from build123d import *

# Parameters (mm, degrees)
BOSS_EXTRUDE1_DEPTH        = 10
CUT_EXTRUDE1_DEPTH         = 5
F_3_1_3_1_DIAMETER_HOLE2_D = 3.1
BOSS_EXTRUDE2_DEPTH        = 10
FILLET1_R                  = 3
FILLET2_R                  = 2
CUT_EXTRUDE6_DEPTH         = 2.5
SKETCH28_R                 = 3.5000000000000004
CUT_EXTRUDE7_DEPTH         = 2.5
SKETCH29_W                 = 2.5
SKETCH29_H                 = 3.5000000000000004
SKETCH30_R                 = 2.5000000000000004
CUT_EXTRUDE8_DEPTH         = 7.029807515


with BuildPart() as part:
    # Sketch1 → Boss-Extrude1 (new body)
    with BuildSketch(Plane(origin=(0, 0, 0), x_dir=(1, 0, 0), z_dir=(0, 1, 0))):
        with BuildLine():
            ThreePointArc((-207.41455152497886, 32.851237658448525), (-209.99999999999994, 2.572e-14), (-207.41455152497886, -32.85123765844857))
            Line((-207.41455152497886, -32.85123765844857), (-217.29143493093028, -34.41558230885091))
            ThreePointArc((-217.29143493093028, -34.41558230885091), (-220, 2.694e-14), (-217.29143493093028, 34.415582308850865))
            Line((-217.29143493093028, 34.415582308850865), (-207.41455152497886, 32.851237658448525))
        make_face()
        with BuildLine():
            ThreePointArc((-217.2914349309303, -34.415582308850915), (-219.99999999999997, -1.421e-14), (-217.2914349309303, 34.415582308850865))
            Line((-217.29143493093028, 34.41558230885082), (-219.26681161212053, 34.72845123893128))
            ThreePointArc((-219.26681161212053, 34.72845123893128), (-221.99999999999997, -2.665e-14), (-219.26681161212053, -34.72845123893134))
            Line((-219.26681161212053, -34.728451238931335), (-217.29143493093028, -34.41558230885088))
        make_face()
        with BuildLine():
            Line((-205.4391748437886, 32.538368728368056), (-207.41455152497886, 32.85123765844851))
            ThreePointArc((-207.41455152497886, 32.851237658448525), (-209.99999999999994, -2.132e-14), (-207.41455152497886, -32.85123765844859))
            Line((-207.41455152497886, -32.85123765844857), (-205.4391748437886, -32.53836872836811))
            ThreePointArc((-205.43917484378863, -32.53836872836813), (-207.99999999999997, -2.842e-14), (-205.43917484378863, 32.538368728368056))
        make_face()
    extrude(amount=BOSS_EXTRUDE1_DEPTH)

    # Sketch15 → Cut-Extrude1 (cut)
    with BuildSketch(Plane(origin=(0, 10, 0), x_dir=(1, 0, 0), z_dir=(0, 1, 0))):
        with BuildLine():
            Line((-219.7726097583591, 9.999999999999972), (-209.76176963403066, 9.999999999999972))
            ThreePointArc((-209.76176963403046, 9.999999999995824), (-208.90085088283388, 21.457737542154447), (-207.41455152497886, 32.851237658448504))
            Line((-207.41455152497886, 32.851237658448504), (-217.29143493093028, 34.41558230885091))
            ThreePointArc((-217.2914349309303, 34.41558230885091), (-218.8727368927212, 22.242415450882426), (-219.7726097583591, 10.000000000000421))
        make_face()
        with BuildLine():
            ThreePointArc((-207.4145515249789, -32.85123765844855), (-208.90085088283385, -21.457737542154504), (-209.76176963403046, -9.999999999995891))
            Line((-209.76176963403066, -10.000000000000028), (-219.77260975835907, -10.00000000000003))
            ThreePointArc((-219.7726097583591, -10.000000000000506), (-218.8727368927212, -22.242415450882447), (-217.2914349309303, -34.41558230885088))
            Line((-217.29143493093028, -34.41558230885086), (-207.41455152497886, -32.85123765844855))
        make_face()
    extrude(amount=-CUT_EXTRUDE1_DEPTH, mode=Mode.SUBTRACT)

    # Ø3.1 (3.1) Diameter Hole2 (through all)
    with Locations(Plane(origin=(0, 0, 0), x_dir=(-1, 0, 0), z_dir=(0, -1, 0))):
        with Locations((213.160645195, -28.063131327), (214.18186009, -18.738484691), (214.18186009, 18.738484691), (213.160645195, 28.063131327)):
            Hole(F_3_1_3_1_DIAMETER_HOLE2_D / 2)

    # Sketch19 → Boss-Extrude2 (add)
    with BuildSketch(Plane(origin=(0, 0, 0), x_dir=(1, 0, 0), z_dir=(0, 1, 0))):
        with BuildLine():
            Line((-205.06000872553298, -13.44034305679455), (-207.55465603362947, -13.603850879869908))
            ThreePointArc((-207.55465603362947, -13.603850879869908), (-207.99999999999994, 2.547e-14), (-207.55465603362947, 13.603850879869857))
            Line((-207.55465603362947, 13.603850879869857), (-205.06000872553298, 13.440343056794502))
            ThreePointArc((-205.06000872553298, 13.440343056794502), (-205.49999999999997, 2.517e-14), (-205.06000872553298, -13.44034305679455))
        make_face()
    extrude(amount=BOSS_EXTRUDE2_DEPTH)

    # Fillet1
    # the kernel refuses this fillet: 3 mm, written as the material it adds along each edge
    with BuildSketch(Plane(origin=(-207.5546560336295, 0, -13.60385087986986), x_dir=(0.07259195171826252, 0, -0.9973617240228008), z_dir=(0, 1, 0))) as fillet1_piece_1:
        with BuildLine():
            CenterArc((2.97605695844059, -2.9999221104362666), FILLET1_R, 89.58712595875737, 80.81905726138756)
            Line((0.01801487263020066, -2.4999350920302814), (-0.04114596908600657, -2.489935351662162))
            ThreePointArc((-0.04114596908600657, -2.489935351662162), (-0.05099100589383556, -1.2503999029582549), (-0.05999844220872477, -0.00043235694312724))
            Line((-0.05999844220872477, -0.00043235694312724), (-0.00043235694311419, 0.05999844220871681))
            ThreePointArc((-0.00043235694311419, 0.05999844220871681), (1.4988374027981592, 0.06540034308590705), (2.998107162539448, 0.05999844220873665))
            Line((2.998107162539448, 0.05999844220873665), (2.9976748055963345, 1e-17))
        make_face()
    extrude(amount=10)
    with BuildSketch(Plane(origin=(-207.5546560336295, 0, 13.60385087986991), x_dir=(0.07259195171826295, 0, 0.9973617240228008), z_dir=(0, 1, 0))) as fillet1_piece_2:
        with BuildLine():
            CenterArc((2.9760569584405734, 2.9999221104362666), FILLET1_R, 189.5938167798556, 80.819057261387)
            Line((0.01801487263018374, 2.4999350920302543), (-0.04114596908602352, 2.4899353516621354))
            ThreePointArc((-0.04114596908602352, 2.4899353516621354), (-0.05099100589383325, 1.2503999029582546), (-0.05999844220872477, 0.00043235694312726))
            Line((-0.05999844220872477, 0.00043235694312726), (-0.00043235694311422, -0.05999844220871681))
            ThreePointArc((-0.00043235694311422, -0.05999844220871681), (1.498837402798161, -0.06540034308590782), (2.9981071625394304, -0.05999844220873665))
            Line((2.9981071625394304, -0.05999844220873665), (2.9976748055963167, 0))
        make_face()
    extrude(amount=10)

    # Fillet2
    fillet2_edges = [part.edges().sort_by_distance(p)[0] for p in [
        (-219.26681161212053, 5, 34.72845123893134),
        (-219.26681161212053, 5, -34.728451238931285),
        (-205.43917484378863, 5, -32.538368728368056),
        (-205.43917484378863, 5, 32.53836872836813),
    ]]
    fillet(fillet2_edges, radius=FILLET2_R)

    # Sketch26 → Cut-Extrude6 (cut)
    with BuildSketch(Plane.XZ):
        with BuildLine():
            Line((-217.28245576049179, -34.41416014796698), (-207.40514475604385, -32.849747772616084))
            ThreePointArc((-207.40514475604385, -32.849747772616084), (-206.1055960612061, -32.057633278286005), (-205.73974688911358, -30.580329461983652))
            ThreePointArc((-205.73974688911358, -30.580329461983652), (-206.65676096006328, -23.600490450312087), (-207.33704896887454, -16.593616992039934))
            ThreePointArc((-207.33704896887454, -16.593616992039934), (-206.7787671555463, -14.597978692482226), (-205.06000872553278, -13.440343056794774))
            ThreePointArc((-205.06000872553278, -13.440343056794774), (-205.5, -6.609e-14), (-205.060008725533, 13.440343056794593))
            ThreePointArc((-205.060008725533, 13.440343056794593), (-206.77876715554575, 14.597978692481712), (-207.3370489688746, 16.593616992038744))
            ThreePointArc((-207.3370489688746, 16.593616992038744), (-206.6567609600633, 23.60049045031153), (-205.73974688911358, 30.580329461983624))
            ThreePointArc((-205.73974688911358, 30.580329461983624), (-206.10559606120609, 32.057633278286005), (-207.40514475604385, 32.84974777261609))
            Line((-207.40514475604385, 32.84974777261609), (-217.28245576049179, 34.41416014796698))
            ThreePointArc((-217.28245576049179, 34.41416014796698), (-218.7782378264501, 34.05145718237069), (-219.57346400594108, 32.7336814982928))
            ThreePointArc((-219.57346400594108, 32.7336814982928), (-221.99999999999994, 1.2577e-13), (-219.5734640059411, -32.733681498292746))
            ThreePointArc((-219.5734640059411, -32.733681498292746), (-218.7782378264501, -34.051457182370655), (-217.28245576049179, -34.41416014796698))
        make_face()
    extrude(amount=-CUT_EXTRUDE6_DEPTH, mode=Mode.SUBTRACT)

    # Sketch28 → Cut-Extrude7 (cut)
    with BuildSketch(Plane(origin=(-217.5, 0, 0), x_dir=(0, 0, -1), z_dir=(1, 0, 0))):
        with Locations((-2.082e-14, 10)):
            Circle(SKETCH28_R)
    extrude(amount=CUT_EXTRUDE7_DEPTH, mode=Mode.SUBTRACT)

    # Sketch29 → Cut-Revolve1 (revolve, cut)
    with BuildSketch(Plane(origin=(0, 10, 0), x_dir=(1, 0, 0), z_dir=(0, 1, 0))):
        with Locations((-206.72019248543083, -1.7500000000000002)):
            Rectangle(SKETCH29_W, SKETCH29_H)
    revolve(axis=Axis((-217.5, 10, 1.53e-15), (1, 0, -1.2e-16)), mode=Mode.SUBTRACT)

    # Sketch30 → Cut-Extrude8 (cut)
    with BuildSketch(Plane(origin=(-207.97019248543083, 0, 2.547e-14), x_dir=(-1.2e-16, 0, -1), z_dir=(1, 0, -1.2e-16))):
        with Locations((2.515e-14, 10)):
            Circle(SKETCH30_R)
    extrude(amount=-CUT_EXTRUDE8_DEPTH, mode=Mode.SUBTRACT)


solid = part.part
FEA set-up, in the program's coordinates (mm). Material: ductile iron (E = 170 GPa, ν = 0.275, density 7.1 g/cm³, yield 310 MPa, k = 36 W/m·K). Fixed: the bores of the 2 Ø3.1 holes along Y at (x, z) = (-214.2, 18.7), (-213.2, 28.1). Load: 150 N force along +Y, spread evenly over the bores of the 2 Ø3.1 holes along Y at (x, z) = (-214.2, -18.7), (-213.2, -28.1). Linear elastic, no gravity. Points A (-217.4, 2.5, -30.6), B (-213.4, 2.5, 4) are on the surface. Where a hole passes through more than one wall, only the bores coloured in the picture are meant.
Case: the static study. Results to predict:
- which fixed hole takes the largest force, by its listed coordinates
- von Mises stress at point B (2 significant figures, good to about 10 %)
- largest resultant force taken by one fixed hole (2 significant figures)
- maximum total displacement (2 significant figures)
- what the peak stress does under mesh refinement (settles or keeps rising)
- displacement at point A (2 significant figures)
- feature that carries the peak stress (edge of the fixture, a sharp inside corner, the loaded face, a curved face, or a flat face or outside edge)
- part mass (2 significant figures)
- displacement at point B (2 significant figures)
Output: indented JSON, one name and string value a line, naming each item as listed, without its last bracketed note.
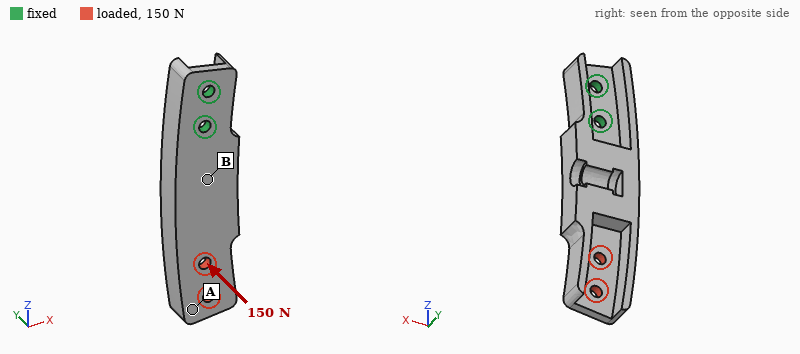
{
  "which fixed hole takes the largest force, by its listed coordinates": "(-214.2, 18.7)",
  "von Mises stress at point B": "34 MPa",
  "largest resultant force taken by one fixed hole": "640 N",
  "maximum total displacement": "0.16 mm",
  "what the peak stress does under mesh refinement": "keeps rising",
  "displacement at point A": "0.15 mm",
  "feature that carries the peak stress": "edge of the fixture",
  "part mass": "35 g",
  "displacement at point B": "0.031 mm"
}
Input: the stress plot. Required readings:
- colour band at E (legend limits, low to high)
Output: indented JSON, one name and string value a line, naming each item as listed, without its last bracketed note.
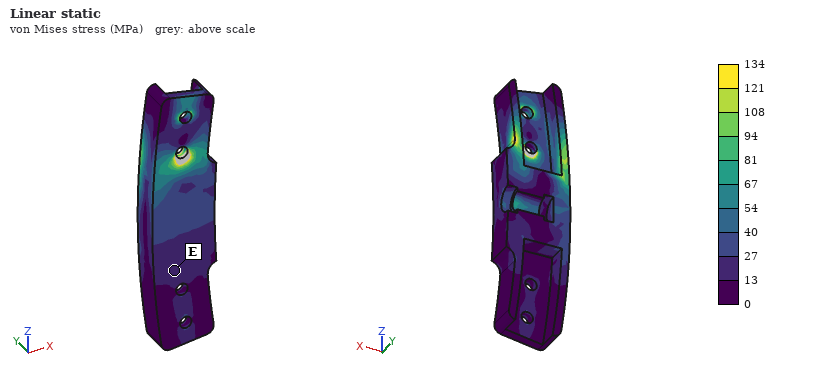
{
  "colour band at E": "13 to 27 MPa"
}
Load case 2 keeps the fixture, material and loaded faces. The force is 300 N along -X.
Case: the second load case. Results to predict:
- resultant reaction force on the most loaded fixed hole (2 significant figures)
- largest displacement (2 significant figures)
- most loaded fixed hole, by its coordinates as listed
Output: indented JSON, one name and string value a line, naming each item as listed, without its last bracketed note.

{
  "resultant reaction force on the most loaded fixed hole": "1.2 kN",
  "largest displacement": "79 µm",
  "most loaded fixed hole, by its coordinates as listed": "(-214.2, 18.7)"
}
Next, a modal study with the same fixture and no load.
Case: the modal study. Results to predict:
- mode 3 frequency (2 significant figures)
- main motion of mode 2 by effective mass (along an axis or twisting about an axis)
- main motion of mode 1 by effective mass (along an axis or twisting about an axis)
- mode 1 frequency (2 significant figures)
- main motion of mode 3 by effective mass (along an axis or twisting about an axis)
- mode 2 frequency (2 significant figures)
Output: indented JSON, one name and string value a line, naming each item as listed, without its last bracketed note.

{
  "mode 3 frequency": "5600 Hz",
  "main motion of mode 2 by effective mass": "along X",
  "main motion of mode 1 by effective mass": "along Y",
  "mode 1 frequency": "1700 Hz",
  "main motion of mode 3 by effective mass": "twisting about Z",
  "mode 2 frequency": "3300 Hz"
}
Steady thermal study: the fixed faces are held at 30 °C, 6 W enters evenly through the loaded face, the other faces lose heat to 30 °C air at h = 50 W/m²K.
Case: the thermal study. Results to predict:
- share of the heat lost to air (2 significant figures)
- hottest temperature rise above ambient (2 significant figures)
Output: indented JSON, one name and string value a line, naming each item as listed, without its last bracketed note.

{
  "share of the heat lost to air": "66 %",
  "hottest temperature rise above ambient": "56 K"
}
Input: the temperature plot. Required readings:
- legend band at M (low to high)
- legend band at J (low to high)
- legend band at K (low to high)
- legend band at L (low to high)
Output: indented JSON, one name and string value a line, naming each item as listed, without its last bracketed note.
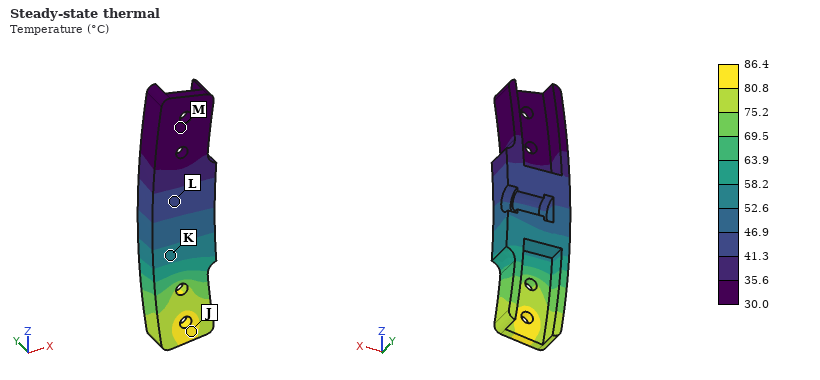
{
  "legend band at M": "30.0 to 35.6 °C",
  "legend band at J": "80.8 to 86.4 °C",
  "legend band at K": "52.6 to 58.2 °C",
  "legend band at L": "41.3 to 46.9 °C"
}
